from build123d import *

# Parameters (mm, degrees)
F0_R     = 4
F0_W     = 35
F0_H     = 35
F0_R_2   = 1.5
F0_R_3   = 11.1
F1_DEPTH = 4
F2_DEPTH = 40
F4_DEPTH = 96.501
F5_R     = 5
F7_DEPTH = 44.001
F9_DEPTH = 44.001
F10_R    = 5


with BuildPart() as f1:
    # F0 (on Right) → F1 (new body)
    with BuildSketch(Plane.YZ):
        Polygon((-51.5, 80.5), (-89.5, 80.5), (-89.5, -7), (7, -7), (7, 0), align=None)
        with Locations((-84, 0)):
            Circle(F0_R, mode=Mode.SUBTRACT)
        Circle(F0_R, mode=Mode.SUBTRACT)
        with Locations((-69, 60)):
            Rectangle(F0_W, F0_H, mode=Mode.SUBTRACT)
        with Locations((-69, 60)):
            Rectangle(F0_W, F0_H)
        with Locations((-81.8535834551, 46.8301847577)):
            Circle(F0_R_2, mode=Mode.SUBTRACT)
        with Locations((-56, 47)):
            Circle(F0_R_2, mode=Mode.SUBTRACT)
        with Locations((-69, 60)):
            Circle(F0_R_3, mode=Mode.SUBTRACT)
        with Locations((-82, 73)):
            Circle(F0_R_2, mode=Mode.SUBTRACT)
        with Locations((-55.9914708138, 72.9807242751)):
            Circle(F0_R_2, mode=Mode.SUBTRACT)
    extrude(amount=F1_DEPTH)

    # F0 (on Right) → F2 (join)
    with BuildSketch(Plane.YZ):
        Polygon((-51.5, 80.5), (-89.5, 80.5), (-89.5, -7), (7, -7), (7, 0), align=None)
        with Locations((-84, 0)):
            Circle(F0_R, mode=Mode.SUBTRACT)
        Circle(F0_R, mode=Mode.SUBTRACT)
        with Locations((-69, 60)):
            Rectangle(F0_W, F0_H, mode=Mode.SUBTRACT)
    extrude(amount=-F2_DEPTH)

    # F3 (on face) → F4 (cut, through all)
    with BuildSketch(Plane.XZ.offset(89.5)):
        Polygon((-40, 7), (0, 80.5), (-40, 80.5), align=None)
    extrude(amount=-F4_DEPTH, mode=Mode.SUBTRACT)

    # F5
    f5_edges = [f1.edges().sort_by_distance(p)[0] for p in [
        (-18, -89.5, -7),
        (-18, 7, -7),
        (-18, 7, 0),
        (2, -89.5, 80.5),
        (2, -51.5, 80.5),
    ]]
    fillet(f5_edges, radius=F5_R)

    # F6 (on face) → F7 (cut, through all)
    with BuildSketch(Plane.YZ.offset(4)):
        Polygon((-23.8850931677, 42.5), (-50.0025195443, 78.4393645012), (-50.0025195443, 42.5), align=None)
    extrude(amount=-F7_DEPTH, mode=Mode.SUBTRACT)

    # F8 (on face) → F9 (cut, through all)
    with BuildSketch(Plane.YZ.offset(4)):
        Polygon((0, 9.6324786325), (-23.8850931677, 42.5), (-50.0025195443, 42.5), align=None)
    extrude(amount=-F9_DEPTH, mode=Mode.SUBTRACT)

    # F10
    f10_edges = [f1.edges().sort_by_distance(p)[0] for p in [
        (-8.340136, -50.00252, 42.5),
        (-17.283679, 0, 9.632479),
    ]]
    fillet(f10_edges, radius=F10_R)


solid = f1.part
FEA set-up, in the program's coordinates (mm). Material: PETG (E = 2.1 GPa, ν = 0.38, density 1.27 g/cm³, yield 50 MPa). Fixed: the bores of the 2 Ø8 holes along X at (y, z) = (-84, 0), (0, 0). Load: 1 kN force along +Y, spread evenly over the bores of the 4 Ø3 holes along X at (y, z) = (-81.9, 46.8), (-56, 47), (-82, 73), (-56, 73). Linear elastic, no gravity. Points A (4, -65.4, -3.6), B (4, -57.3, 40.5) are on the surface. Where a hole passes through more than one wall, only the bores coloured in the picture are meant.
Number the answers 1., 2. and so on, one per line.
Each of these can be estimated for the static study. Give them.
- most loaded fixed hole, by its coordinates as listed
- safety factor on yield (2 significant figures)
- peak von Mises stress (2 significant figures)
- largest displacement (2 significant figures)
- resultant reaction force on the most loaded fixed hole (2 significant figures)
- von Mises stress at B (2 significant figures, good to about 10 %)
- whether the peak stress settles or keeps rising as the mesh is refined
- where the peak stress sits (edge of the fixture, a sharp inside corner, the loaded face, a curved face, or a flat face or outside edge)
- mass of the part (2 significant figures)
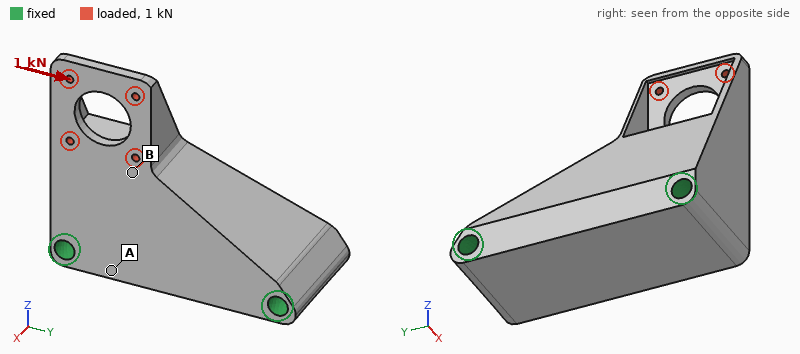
1. (0, 0)
2. 1.2
3. 40 MPa
4. 1.2 mm
5. 1.1 kN
6. 4.6 MPa
7. settles
8. a curved face
9. 180 g
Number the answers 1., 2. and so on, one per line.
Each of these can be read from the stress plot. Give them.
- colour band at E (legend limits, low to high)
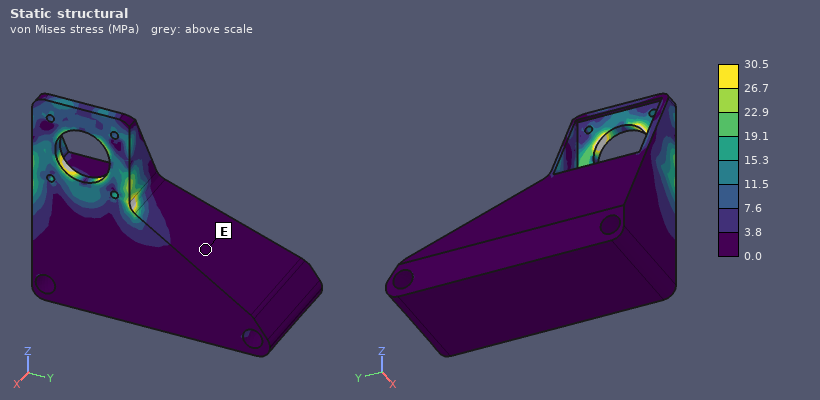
1. 0.0 to 3.8 MPa
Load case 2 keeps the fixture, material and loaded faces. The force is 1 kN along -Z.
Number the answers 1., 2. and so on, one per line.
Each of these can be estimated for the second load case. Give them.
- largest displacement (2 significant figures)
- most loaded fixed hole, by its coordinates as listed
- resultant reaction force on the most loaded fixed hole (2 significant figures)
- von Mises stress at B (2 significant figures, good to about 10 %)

1. 0.45 mm
2. (-84, 0)
3. 850 N
4. 7.1 MPa
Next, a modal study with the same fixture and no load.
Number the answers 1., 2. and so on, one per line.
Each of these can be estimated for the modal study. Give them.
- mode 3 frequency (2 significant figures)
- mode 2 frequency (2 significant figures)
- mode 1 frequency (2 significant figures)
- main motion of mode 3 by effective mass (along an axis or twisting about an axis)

1. 2300 Hz
2. 1800 Hz
3. 1400 Hz
4. along X
